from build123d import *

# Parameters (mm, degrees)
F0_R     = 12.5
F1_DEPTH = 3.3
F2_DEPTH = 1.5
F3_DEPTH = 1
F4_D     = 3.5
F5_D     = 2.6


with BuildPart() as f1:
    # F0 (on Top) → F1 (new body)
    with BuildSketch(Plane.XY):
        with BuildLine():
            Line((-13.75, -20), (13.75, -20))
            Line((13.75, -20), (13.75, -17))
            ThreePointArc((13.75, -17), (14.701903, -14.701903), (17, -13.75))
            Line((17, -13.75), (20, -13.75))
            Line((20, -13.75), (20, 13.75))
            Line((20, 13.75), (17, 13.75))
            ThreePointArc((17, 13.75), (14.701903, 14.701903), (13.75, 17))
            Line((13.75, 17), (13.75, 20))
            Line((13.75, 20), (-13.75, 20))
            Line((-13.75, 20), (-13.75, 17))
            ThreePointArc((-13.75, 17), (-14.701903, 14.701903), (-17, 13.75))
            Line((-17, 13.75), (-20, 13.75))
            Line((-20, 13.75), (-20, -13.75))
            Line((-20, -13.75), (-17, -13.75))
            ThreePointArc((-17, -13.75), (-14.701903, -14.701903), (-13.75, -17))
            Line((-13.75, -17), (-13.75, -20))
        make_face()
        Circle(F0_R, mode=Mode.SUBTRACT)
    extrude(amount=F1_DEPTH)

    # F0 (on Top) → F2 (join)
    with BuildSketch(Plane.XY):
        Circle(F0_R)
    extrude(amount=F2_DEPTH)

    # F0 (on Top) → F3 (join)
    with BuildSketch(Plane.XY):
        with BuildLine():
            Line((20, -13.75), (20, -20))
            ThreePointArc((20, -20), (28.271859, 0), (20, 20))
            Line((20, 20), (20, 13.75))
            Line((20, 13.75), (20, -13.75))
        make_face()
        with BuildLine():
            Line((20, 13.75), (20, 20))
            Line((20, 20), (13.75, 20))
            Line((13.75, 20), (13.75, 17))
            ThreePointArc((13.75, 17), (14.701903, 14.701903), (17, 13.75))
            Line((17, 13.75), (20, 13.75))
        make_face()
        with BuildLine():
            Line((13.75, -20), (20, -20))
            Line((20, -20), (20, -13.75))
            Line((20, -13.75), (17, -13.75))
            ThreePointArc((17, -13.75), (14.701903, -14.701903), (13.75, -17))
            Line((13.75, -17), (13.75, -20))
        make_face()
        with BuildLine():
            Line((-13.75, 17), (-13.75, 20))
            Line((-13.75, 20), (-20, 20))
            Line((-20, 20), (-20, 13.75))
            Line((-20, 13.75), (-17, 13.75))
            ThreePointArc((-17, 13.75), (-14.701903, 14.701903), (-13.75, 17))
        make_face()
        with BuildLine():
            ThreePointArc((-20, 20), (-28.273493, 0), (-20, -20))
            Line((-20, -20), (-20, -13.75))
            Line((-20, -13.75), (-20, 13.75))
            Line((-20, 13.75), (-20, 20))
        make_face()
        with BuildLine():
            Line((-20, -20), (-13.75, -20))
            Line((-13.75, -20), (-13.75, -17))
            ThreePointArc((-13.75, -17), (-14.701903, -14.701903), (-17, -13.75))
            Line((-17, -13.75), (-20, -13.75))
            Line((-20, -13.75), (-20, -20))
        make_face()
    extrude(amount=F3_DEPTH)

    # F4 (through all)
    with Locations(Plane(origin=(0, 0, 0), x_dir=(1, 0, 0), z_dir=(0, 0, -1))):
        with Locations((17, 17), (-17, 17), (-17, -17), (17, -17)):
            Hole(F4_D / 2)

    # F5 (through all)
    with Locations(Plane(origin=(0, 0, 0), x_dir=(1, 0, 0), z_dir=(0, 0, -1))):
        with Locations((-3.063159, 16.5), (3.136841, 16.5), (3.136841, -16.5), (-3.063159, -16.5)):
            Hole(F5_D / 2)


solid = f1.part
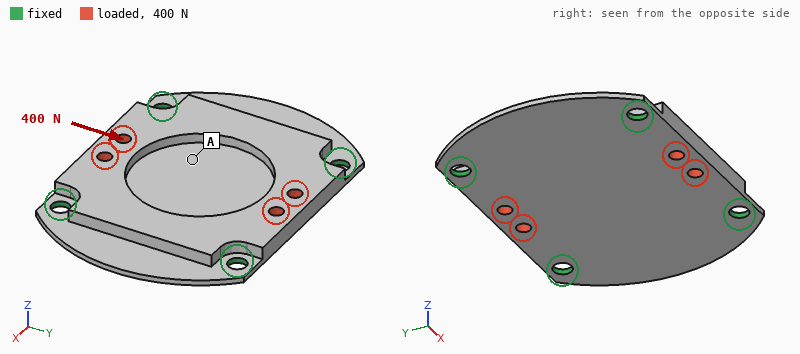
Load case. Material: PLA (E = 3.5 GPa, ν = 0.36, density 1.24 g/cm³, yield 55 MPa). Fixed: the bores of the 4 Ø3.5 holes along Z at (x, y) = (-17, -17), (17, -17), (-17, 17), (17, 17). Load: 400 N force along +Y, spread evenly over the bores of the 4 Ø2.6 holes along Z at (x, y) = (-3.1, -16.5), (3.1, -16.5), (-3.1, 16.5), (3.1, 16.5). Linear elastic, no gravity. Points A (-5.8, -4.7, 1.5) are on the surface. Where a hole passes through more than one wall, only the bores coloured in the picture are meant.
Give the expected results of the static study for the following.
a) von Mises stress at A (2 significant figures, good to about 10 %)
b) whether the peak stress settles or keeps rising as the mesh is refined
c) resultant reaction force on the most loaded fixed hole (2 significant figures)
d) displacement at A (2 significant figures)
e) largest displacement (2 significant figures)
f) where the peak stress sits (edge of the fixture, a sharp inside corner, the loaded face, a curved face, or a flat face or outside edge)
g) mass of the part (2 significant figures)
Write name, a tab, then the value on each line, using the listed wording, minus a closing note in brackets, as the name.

von Mises stress at A	4.2 MPa
whether the peak stress settles or keeps rising as the mesh is refined	keeps rising
resultant reaction force on the most loaded fixed hole	100 N
displacement at A	33 µm
largest displacement	59 µm
where the peak stress sits	edge of the fixture
mass of the part	5.5 g
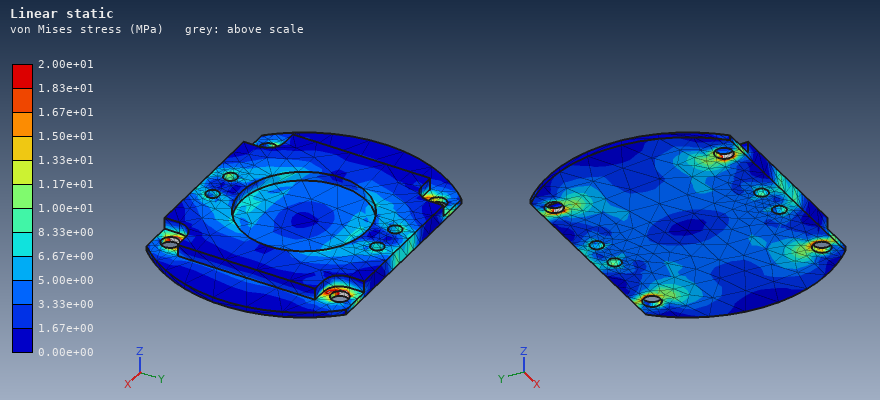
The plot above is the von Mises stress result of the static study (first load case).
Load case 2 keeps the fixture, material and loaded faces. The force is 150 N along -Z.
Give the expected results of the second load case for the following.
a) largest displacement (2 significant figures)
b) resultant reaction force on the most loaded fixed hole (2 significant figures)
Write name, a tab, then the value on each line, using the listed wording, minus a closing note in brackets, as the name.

largest displacement	0.30 mm
resultant reaction force on the most loaded fixed hole	92 N
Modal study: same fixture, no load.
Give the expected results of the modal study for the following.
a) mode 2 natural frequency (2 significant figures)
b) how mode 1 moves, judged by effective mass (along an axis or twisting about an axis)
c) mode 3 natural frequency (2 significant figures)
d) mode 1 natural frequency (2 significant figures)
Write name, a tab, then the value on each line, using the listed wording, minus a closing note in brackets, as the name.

mode 2 natural frequency	2900 Hz
how mode 1 moves, judged by effective mass	along Z
mode 3 natural frequency	3000 Hz
mode 1 natural frequency	2300 Hz
